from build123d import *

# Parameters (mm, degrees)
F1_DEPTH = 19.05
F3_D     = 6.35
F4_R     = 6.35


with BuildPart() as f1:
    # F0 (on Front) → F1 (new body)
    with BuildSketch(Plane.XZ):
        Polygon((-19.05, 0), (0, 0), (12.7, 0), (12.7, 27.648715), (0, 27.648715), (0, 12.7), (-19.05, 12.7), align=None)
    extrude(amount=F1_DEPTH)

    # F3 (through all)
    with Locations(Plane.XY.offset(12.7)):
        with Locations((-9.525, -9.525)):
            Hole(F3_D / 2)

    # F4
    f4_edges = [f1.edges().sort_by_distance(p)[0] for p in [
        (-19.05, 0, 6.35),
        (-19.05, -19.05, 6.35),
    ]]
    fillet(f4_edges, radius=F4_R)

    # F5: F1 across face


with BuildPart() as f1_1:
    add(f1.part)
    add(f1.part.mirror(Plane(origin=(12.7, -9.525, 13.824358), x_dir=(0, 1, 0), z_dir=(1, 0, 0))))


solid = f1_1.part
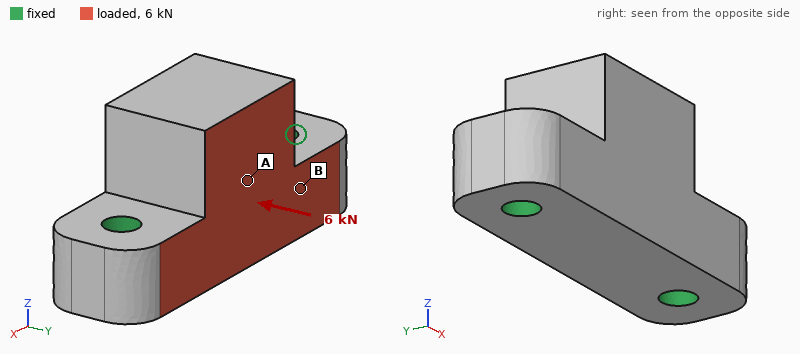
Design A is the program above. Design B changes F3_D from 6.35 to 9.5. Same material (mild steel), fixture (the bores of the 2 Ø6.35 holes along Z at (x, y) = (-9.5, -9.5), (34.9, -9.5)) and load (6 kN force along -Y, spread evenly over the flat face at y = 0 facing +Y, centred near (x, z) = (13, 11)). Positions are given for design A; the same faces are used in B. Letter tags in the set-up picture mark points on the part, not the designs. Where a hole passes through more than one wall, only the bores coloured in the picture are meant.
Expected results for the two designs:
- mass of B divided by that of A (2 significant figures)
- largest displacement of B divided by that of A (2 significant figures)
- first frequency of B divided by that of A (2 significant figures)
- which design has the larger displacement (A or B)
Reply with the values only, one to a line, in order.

0.95
0.80
1.1
A
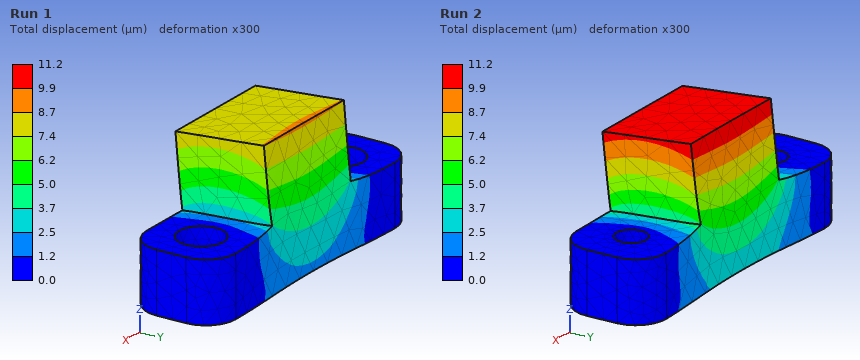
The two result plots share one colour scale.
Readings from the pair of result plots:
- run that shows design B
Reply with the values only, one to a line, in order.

Run 1
